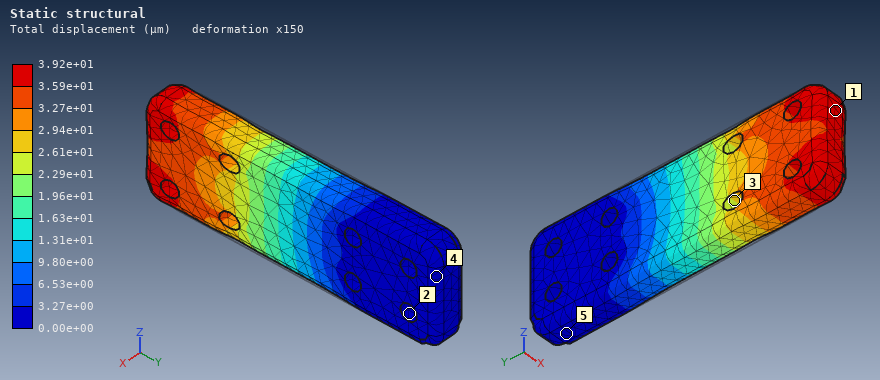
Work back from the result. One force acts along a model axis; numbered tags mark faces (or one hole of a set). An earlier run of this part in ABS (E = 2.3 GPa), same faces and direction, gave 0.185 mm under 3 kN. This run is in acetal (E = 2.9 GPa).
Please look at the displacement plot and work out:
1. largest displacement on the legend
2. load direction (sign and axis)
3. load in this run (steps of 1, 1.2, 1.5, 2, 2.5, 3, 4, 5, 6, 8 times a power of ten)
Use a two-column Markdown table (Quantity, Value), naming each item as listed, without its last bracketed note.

| Quantity | Value |
|---|---|
| largest displacement on the legend | 3.92e+01 µm |
| load direction | -Y |
| load in this run | 800 N |
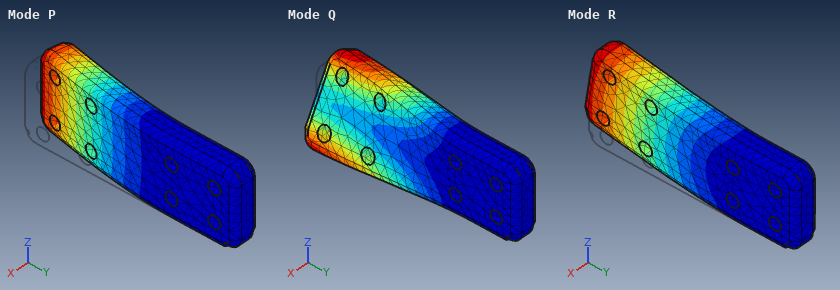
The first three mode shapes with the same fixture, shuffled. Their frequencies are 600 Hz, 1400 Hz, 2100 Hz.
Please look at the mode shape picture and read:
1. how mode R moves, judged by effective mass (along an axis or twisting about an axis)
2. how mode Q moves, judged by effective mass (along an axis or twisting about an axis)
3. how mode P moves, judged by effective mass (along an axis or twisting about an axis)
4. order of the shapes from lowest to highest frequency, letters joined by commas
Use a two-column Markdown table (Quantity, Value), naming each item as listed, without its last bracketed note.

| Quantity | Value |
|---|---|
| how mode R moves, judged by effective mass | along Z |
| how mode Q moves, judged by effective mass | twisting about Y |
| how mode P moves, judged by effective mass | along X |
| order of the shapes from lowest to highest frequency, letters joined by commas | P, R, Q |
